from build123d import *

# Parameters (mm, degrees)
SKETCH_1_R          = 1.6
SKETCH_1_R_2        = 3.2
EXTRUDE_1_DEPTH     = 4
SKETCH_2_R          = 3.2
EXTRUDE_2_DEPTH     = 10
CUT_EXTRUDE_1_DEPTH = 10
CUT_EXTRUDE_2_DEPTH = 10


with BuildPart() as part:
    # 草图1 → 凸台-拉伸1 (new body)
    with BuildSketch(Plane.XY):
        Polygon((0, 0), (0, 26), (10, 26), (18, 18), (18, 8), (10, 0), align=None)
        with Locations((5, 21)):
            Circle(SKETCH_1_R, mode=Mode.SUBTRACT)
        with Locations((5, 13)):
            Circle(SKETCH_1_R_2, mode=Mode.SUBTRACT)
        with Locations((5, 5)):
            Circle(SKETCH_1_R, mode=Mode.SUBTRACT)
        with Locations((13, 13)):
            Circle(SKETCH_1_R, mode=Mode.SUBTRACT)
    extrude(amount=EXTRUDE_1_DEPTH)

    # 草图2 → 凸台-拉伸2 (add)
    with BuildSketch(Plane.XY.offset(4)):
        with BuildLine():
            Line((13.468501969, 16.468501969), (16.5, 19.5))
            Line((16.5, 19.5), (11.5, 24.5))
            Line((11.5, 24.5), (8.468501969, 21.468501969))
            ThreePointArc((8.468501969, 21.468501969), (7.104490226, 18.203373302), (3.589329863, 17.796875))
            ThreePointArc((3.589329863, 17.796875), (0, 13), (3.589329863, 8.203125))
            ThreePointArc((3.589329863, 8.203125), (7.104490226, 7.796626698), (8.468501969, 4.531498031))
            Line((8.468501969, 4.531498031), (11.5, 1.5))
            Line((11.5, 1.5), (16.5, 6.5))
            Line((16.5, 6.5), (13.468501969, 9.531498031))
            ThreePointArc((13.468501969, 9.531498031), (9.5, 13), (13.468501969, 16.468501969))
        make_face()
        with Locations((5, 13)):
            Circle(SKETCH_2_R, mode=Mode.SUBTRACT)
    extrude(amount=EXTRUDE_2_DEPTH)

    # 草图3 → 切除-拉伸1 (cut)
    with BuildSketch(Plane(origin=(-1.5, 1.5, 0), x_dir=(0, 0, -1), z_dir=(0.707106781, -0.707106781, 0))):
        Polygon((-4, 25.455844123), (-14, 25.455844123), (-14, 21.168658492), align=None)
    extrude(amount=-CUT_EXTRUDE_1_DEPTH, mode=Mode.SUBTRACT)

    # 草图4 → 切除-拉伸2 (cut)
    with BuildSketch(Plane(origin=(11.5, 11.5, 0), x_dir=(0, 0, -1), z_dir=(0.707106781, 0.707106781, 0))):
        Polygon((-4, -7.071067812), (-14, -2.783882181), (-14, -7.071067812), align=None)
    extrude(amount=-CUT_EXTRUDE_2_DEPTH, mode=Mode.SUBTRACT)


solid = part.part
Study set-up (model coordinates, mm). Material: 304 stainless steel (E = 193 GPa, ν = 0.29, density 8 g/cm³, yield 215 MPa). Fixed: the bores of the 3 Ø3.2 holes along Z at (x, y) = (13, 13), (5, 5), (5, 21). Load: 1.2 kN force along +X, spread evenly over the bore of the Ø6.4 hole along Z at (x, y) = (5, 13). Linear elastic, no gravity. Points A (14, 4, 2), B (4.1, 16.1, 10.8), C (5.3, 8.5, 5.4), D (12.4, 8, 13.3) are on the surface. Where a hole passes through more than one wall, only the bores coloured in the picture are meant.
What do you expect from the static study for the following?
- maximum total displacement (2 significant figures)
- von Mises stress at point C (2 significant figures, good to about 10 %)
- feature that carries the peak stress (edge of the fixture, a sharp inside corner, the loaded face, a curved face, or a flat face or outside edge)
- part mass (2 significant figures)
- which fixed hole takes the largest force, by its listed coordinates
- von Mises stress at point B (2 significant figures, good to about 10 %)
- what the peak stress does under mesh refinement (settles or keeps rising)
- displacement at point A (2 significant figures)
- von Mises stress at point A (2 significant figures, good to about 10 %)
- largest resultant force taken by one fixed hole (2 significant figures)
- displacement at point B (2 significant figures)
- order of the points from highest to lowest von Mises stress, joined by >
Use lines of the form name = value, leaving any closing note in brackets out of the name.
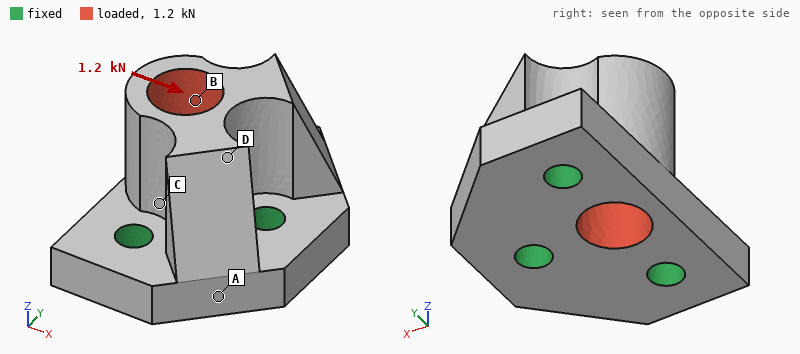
maximum total displacement = 4.6 µm
von Mises stress at point C = 37 MPa
feature that carries the peak stress = edge of the fixture
part mass = 20 g
which fixed hole takes the largest force, by its listed coordinates = (13, 13)
von Mises stress at point B = 25 MPa
what the peak stress does under mesh refinement = keeps rising
displacement at point A = 1.2 µm
von Mises stress at point A = 12 MPa
largest resultant force taken by one fixed hole = 690 N
displacement at point B = 3.3 µm
order of the points from highest to lowest von Mises stress, joined by > = C > B > A > D
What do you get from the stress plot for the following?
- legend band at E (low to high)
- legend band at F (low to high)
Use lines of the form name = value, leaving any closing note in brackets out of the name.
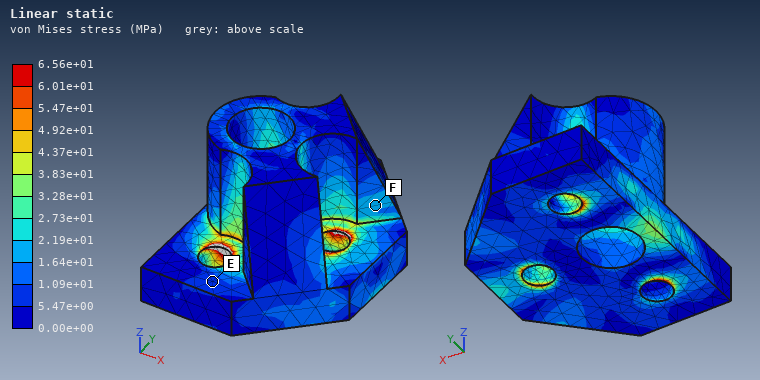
legend band at E = 5.47e+00 to 1.09e+01 MPa
legend band at F = 1.64e+01 to 2.19e+01 MPa
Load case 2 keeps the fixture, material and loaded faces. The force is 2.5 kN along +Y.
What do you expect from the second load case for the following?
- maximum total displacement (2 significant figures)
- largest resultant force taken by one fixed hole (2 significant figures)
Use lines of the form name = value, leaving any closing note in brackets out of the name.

maximum total displacement = 8.7 µm
largest resultant force taken by one fixed hole = 1.2 kN
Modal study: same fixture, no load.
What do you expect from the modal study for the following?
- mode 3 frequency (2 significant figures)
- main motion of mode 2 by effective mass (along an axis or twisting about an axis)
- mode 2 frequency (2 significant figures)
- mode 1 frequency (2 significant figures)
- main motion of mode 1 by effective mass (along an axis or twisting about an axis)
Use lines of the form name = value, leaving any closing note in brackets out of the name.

mode 3 frequency = 49 kHz
main motion of mode 2 by effective mass = along Y
mode 2 frequency = 36 kHz
mode 1 frequency = 30 kHz
main motion of mode 1 by effective mass = along X
